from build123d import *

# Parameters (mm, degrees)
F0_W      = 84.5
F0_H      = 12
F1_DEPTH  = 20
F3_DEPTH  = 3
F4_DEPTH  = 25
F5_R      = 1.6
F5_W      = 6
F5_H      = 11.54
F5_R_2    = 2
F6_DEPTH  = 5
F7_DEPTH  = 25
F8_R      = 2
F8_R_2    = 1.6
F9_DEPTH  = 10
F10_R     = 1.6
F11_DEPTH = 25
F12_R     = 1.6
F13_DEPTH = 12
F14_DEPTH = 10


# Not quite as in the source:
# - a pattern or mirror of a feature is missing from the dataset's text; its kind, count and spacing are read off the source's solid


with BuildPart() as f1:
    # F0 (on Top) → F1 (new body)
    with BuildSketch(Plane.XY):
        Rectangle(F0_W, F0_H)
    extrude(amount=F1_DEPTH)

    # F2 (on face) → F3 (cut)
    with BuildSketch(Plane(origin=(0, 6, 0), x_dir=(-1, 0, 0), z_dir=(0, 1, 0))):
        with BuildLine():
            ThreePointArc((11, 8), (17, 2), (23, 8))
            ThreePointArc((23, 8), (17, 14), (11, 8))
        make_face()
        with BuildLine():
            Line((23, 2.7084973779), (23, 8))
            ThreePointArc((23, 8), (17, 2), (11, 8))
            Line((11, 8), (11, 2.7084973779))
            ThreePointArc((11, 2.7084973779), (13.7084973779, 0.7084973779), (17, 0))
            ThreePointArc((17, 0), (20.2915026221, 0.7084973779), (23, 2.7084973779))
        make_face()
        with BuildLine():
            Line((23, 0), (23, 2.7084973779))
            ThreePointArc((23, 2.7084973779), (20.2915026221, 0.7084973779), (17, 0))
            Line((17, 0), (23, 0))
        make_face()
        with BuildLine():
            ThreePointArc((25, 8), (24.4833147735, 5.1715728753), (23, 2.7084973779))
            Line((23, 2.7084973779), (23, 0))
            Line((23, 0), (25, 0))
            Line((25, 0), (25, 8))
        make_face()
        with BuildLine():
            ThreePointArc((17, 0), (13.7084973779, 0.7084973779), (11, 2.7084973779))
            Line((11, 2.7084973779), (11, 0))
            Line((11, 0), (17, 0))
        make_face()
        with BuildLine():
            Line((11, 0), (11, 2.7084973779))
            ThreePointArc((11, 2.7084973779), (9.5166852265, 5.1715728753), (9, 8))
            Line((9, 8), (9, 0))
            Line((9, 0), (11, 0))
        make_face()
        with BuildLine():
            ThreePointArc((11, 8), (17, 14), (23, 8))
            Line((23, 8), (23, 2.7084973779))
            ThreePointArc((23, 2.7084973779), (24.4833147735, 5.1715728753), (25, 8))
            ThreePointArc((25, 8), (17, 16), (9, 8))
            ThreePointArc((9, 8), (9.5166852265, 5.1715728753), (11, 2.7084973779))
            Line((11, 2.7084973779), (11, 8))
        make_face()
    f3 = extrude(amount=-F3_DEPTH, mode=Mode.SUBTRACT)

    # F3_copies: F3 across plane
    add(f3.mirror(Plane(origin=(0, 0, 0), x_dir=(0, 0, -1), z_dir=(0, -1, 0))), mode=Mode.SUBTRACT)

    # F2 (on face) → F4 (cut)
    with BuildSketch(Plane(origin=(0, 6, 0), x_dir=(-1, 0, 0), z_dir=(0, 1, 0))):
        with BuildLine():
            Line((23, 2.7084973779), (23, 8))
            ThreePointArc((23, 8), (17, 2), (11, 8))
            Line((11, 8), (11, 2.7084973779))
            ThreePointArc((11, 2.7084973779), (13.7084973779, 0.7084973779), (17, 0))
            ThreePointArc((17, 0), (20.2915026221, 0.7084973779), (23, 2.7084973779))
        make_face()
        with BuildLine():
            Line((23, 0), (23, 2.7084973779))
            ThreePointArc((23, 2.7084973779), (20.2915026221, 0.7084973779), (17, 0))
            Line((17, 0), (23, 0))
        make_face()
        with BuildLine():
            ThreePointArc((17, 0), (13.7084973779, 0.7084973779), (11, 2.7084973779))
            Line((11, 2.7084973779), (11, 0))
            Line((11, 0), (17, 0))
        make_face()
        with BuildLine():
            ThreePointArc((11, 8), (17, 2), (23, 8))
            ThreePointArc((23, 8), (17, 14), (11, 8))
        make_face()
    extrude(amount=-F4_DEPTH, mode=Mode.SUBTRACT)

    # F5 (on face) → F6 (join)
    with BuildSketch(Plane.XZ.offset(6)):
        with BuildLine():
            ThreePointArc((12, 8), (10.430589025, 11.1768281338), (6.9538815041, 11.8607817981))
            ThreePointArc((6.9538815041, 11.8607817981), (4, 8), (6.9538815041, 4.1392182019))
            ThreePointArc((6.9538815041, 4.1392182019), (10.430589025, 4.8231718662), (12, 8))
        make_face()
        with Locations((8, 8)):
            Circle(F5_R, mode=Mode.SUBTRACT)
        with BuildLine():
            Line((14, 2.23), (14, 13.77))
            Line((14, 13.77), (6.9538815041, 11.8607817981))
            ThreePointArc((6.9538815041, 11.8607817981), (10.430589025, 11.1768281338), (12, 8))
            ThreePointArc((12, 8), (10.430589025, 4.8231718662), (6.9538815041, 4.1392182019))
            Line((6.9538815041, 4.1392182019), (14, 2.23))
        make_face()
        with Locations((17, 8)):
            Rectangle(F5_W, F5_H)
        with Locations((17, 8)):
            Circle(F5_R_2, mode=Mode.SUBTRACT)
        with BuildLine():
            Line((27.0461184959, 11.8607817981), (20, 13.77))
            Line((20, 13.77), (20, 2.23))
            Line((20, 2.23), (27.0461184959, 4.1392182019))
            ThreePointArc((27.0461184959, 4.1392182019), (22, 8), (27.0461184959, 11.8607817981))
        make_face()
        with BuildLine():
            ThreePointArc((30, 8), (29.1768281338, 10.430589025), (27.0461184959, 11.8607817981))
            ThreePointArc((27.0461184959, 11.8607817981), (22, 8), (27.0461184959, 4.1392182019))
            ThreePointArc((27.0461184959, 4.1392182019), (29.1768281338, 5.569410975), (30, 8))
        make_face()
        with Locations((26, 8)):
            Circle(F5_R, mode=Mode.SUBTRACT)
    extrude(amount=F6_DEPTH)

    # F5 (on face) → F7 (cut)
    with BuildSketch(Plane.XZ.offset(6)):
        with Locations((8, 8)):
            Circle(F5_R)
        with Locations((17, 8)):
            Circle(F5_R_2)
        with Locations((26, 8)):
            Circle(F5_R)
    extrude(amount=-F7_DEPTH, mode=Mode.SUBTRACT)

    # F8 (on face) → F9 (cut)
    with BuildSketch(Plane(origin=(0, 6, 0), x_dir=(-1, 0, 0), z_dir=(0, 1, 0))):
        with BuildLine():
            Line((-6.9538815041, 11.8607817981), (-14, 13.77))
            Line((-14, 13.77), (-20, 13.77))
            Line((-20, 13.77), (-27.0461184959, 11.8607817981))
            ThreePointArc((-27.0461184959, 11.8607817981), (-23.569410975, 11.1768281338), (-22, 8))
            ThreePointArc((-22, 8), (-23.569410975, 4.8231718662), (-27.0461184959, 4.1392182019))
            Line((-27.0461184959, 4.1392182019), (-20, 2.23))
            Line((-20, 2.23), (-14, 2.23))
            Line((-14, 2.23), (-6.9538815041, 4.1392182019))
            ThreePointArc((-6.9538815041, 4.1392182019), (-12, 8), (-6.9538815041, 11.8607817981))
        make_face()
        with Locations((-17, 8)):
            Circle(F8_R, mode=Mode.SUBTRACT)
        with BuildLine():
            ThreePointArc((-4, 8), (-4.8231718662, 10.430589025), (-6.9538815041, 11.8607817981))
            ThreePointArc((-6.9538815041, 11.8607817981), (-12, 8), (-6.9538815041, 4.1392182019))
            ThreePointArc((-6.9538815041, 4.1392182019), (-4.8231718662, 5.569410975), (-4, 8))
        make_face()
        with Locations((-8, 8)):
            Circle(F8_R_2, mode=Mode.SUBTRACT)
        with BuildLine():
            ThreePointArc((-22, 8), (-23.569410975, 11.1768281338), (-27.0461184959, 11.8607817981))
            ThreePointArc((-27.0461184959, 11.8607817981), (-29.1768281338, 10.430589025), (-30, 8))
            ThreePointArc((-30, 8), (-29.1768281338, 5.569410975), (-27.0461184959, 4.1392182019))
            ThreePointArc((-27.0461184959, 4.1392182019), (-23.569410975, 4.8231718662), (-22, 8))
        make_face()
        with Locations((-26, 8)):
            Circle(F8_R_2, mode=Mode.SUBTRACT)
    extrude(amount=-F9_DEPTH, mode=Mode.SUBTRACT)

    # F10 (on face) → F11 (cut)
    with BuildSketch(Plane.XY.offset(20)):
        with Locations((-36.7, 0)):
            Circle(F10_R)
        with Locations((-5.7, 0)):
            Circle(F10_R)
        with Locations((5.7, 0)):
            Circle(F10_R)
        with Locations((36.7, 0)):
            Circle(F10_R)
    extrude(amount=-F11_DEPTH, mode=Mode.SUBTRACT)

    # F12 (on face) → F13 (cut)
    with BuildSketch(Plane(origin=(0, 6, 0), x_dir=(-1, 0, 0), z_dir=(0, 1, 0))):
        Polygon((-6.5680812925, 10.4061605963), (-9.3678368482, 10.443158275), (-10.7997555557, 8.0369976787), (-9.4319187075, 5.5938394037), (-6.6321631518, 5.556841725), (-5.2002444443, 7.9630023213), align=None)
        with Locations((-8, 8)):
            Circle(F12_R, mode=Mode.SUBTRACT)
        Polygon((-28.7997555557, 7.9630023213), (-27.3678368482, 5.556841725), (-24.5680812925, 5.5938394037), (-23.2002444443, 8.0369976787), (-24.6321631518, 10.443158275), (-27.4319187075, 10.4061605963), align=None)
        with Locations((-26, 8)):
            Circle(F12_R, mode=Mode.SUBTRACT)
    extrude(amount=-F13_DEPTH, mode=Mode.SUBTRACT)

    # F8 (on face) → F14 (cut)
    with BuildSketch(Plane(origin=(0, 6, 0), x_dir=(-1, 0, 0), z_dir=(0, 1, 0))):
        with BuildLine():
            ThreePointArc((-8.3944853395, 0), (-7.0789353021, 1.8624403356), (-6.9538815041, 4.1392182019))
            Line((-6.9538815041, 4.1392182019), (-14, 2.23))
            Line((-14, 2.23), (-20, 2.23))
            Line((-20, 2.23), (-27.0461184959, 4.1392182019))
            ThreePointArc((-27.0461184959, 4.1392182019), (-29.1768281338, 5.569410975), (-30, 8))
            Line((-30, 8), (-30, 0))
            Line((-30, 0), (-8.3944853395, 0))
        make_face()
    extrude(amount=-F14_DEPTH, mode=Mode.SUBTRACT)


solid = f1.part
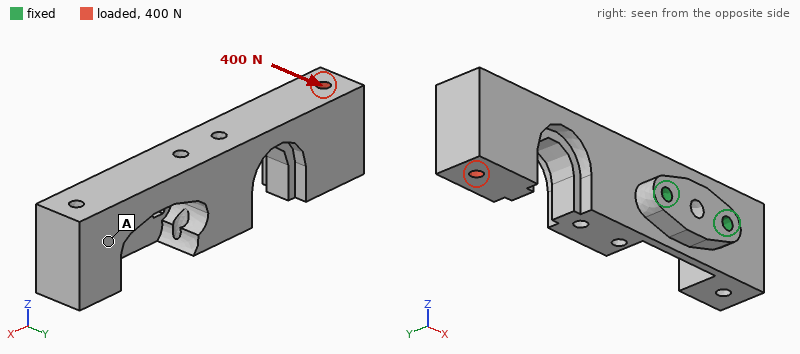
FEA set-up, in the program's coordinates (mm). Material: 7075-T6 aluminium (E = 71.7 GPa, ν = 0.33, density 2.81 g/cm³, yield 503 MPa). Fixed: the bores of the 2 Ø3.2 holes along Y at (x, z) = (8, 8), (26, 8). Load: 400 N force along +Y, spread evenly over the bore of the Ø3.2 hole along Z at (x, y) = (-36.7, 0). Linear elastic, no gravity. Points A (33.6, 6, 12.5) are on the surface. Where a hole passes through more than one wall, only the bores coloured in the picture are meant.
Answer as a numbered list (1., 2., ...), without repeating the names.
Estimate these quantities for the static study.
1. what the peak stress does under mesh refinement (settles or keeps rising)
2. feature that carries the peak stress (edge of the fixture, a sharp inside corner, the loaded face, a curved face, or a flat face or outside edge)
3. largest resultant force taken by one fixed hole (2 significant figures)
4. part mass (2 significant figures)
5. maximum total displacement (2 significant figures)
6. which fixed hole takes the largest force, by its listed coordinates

1. keeps rising
2. a sharp inside corner
3. 1.3 kN
4. 43 g
5. 0.36 mm
6. (8, 8)
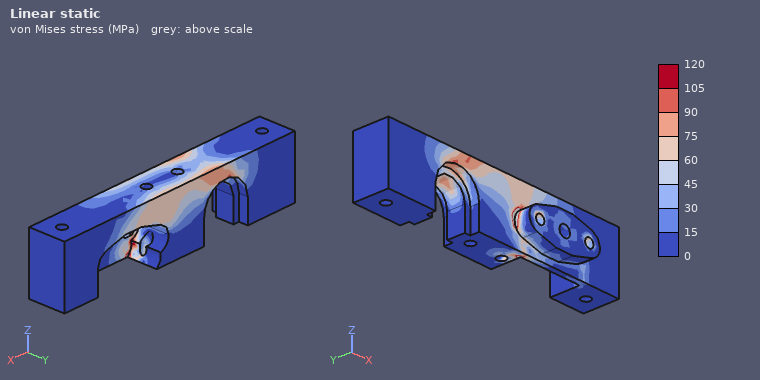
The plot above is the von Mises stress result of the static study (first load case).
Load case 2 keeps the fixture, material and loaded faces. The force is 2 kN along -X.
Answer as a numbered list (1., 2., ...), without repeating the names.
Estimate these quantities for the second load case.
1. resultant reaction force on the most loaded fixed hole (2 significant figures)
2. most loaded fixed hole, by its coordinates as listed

1. 1.4 kN
2. (8, 8)
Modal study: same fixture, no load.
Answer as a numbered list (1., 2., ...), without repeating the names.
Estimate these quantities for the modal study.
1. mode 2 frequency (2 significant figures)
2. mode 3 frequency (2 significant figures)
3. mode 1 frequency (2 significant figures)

1. 2100 Hz
2. 4300 Hz
3. 1600 Hz
